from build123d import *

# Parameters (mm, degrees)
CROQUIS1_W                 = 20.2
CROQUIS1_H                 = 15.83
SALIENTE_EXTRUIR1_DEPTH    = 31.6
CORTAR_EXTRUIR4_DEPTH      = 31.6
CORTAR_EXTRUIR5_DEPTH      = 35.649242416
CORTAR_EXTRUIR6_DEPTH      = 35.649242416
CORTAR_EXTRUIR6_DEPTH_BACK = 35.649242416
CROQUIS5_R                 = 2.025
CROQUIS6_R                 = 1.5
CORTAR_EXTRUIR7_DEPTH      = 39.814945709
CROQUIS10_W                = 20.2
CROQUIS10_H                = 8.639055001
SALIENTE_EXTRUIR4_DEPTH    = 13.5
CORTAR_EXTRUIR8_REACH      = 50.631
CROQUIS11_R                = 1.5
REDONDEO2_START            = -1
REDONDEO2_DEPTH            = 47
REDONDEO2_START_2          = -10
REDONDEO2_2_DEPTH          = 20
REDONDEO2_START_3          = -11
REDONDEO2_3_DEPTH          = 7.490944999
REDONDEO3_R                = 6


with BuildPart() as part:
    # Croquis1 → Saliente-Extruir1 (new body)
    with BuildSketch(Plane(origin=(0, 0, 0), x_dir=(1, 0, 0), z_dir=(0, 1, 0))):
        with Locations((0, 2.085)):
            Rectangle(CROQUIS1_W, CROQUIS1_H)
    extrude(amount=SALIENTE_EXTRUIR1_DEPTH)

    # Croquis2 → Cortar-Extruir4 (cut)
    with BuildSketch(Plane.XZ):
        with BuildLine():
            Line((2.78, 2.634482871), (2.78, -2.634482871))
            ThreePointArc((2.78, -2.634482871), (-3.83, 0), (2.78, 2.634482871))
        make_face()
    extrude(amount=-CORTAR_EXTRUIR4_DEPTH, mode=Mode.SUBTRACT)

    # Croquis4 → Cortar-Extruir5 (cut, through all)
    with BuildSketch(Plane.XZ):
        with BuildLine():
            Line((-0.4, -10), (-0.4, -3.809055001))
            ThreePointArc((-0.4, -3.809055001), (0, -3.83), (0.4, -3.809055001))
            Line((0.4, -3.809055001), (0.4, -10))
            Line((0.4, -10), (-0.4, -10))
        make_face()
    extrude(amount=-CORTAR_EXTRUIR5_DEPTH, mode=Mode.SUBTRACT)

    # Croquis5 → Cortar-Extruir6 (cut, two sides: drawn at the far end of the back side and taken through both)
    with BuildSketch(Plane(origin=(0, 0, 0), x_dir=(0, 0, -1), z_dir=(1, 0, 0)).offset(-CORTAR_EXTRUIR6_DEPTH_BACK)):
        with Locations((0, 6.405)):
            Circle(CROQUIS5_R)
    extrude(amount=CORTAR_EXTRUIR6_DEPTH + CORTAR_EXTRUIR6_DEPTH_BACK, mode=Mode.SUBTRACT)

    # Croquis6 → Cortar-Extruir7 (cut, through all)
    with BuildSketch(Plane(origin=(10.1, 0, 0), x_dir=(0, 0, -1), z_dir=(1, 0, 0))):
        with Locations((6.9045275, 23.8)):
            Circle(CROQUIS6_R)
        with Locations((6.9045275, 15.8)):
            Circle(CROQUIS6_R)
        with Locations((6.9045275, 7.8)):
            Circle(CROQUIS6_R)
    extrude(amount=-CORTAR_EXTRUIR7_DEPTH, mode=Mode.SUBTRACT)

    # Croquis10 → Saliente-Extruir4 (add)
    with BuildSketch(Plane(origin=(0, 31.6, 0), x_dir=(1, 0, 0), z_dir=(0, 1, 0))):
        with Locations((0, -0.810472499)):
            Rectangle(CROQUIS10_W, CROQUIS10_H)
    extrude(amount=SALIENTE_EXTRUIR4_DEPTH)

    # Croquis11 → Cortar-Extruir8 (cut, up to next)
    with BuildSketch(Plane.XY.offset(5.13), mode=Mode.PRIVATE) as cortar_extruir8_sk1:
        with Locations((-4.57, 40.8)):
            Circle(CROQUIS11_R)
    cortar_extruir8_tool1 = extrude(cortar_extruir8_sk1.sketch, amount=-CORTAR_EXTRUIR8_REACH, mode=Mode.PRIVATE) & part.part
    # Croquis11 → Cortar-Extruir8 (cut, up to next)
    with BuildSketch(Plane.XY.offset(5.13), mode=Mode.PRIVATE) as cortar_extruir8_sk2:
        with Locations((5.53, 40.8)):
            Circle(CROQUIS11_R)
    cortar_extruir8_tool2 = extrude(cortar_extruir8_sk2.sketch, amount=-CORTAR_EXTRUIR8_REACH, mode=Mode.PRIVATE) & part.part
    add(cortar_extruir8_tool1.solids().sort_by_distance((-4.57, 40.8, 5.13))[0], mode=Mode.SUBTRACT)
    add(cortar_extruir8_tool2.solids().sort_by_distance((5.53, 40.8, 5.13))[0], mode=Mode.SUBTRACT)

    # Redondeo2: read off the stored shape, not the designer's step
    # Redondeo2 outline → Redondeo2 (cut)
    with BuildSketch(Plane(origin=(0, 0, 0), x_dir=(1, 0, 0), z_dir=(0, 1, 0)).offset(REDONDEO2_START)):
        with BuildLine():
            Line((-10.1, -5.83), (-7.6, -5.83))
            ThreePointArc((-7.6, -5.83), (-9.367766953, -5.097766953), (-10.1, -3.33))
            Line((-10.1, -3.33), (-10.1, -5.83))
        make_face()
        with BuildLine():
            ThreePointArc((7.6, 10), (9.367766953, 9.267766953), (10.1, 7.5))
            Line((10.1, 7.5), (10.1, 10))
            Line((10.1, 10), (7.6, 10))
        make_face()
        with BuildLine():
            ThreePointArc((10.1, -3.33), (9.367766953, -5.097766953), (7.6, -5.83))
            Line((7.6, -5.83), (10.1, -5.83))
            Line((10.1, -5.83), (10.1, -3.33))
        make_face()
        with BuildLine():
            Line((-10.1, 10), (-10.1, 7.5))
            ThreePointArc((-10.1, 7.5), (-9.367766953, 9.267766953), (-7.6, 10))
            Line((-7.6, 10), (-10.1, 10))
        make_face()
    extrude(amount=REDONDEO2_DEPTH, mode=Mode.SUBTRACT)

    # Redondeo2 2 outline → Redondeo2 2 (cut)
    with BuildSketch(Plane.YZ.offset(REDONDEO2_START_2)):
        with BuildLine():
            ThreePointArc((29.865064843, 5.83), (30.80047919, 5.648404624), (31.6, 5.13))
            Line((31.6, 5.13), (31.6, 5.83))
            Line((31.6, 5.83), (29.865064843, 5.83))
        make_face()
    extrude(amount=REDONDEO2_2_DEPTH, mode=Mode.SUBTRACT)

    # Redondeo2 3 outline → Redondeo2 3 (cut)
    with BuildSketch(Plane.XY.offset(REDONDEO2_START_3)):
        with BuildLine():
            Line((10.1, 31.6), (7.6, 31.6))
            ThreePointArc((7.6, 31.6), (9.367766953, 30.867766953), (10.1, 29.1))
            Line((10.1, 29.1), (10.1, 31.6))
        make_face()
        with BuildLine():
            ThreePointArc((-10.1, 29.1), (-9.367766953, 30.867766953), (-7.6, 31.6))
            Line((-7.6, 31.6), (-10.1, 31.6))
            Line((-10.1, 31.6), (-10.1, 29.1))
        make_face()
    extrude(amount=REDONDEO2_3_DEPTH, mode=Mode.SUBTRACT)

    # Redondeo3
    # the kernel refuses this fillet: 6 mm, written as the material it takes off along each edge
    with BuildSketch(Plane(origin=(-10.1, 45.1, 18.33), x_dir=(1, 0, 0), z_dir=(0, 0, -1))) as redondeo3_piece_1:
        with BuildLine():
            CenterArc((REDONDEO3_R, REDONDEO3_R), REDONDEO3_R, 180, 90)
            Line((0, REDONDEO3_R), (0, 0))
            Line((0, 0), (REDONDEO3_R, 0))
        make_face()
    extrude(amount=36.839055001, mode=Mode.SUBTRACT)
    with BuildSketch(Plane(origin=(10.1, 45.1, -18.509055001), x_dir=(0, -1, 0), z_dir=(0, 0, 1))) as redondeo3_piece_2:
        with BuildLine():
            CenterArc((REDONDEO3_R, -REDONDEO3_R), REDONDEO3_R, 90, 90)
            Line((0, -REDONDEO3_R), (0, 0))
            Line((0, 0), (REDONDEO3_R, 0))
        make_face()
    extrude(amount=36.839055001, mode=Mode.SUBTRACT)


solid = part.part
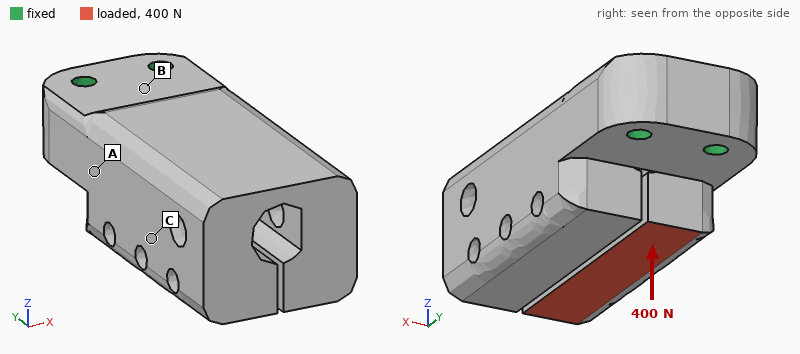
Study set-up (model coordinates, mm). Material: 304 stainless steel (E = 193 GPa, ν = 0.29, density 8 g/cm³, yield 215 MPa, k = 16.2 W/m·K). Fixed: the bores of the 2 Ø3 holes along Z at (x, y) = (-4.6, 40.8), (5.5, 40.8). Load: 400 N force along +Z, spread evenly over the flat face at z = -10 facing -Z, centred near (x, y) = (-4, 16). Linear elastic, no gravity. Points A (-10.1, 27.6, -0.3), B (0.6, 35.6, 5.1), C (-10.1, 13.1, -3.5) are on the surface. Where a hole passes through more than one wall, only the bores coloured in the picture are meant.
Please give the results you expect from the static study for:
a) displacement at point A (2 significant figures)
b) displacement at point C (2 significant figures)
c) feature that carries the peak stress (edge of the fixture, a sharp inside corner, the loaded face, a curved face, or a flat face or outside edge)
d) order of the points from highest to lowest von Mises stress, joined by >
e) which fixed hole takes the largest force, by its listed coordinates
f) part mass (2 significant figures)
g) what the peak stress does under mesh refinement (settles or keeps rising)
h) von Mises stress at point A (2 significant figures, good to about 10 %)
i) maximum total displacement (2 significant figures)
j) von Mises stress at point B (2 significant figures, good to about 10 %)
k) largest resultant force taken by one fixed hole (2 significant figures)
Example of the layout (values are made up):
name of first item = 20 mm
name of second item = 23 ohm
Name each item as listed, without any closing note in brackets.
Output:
displacement at point A = 4.8 µm
displacement at point C = 14 µm
feature that carries the peak stress = edge of the fixture
order of the points from highest to lowest von Mises stress, joined by > = B > A > C
which fixed hole takes the largest force, by its listed coordinates = (-4.6, 40.8)
part mass = 79 g
what the peak stress does under mesh refinement = keeps rising
von Mises stress at point A = 11 MPa
maximum total displacement = 23 µm
von Mises stress at point B = 26 MPa
largest resultant force taken by one fixed hole = 300 N
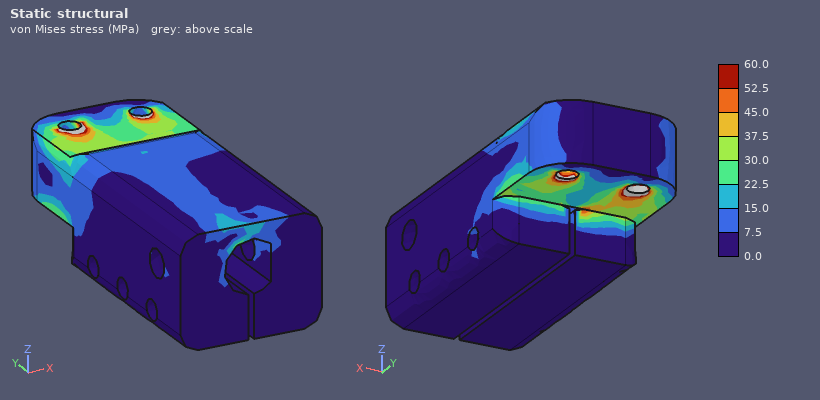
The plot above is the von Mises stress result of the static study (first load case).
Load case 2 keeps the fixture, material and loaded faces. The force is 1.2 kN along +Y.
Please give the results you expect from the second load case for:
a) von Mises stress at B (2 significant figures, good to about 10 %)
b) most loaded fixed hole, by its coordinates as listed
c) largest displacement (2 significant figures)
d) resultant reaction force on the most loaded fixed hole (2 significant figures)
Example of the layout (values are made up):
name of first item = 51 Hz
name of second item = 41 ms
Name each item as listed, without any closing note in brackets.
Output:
von Mises stress at B = 38 MPa
most loaded fixed hole, by its coordinates as listed = (-4.6, 40.8)
largest displacement = 41 µm
resultant reaction force on the most loaded fixed hole = 1.1 kN
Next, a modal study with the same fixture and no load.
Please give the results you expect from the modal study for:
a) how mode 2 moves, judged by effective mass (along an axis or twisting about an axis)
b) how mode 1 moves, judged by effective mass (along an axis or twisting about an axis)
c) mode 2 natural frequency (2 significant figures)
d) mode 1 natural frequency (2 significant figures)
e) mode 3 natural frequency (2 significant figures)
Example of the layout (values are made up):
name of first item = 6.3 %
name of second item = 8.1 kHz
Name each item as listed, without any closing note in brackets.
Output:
how mode 2 moves, judged by effective mass = along X
how mode 1 moves, judged by effective mass = along Z
mode 2 natural frequency = 5000 Hz
mode 1 natural frequency = 3400 Hz
mode 3 natural frequency = 9100 Hz
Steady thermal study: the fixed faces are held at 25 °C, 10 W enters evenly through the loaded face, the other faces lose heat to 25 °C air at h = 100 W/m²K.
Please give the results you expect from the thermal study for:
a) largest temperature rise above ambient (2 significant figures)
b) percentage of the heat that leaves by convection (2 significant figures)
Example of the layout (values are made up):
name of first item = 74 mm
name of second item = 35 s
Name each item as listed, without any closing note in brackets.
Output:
largest temperature rise above ambient = 54 K
percentage of the heat that leaves by convection = 74 %
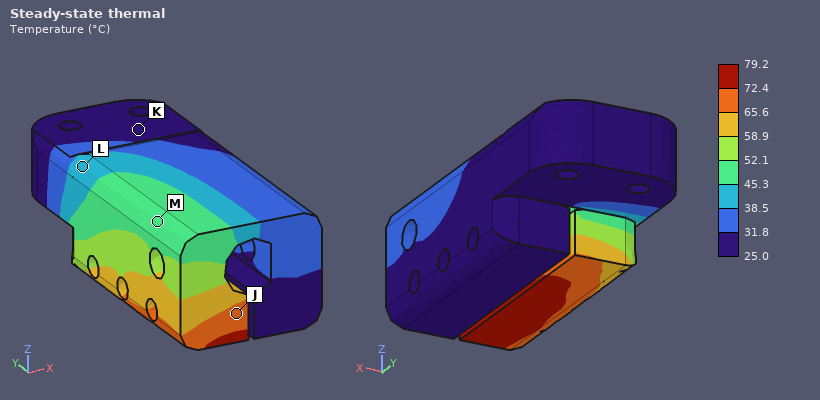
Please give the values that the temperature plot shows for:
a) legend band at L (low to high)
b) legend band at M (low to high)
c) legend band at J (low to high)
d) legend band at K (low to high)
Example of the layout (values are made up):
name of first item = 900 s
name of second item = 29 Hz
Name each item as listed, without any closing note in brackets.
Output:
legend band at L = 38.5 to 45.3 °C
legend band at M = 45.3 to 52.1 °C
legend band at J = 65.6 to 72.4 °C
legend band at K = 25.0 to 31.8 °C
